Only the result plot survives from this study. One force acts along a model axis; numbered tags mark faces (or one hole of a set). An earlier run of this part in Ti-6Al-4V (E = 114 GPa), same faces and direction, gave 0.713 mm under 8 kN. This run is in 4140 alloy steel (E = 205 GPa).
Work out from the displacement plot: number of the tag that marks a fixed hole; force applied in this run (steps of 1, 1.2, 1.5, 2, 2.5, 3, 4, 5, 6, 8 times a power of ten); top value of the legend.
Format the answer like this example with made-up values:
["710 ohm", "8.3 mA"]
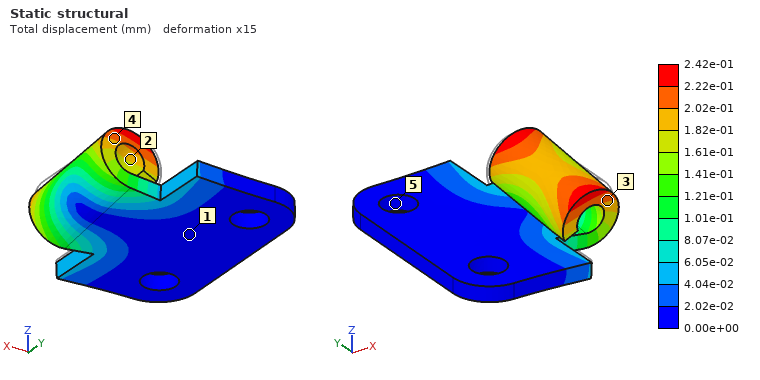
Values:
["5", "5 kN", "2.42e-01 mm"]
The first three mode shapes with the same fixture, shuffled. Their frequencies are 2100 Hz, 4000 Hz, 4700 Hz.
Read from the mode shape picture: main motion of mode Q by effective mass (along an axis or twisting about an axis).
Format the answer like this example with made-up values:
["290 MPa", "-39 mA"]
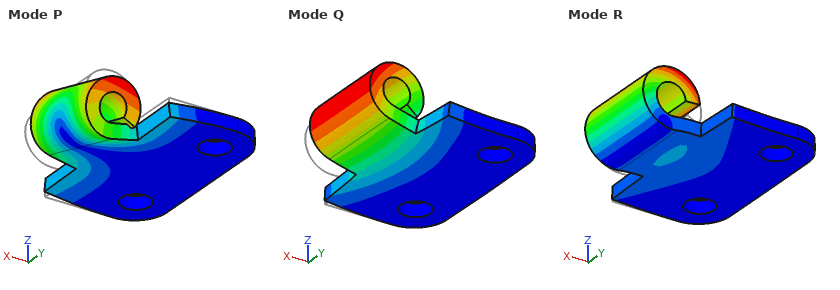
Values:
["along Z"]
